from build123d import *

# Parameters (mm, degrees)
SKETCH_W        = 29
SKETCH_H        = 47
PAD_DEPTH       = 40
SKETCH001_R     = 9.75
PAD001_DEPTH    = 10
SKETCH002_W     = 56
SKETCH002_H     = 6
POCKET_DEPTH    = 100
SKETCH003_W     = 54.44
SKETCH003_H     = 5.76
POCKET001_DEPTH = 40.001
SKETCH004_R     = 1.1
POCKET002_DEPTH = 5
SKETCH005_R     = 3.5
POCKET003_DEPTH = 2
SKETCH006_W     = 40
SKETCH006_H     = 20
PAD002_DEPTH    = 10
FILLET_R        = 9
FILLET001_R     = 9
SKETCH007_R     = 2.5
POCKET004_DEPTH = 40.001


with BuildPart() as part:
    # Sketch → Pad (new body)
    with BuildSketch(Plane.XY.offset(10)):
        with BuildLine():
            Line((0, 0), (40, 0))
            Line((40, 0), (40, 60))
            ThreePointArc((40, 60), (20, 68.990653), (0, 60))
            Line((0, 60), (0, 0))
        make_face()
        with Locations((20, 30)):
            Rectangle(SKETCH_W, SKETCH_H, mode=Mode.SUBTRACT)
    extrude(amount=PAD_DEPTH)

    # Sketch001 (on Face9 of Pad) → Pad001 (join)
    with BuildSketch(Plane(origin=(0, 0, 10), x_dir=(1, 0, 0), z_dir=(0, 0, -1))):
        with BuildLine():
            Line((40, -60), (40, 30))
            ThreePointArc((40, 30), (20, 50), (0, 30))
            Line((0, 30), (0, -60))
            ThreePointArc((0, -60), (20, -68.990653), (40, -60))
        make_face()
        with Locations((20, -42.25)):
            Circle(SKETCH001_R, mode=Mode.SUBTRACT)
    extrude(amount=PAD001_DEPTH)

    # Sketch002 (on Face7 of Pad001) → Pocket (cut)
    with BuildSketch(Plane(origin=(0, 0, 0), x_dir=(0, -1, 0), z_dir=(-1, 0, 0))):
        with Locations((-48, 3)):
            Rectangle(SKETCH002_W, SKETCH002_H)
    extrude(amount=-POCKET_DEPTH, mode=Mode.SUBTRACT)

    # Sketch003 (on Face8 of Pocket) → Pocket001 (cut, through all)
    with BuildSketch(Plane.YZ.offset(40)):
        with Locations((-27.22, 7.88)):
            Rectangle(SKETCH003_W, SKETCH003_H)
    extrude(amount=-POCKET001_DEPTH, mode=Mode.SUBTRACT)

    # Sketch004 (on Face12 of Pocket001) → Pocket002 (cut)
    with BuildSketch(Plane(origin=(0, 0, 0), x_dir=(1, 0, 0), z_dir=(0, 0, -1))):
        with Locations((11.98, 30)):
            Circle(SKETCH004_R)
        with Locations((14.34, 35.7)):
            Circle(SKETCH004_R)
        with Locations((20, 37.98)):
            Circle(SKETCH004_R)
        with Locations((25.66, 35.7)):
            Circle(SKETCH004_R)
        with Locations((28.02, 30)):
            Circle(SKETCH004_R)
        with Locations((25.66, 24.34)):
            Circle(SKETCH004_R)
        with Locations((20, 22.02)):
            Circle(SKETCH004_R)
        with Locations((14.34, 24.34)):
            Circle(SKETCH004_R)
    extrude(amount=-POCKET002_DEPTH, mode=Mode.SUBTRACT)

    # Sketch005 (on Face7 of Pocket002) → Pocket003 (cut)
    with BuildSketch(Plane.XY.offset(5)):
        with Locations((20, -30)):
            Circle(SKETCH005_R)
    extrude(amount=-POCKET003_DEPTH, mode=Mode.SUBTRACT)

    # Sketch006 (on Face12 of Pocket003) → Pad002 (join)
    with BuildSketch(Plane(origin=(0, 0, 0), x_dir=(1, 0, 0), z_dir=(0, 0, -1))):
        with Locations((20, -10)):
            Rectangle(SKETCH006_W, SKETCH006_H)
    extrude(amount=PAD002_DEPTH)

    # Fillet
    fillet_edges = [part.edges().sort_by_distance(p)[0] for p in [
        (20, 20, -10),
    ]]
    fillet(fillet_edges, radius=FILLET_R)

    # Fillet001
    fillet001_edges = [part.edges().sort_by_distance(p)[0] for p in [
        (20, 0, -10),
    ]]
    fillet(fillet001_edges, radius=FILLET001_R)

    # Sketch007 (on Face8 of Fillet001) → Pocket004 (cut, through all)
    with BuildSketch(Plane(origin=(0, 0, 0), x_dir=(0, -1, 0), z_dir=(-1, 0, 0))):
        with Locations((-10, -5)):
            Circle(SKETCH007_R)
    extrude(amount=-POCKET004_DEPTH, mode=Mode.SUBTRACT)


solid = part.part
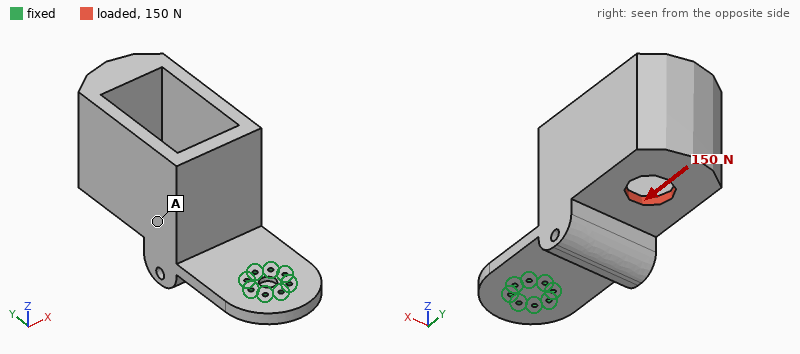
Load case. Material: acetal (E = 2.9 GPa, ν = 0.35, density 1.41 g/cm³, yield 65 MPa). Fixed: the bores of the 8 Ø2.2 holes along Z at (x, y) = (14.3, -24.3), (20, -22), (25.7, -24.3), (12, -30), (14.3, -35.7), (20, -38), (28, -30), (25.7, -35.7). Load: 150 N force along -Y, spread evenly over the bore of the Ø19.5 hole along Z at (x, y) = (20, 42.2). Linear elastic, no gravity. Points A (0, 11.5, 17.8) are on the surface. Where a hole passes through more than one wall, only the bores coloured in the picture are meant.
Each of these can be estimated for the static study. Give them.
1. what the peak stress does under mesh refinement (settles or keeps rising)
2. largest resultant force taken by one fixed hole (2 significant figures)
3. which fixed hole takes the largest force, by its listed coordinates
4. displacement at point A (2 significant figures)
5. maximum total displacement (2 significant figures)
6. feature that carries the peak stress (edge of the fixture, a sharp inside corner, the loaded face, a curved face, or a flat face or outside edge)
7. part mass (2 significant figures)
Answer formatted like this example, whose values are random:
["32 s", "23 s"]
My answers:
["keeps rising", "47 N", "(20, -22)", "0.46 mm", "1.5 mm", "edge of the fixture", "110 g"]
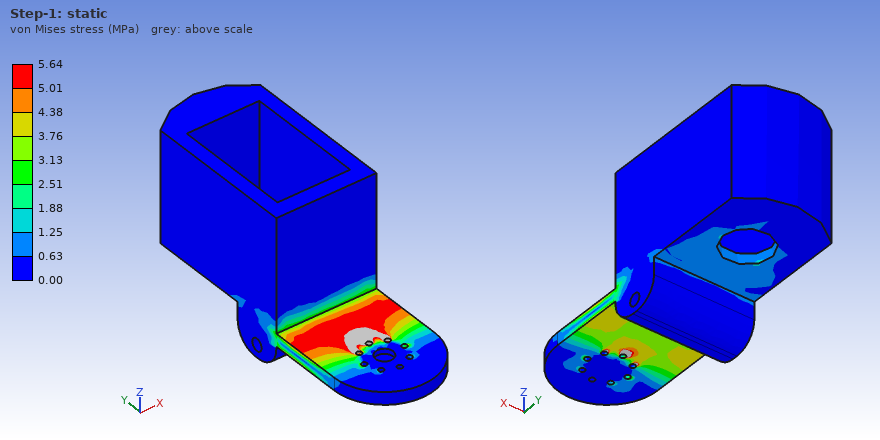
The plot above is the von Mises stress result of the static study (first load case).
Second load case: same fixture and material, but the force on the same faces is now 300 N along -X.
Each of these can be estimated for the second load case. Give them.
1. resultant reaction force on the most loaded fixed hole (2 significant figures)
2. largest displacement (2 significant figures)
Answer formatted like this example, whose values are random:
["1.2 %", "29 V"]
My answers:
["430 N", "1.6 mm"]
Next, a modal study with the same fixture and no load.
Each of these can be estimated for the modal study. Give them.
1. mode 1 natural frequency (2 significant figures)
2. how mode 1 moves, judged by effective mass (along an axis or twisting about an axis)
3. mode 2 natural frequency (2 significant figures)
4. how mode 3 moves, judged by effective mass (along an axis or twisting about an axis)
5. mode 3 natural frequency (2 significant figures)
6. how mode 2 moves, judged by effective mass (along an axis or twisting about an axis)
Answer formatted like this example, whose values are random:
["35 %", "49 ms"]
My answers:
["63 Hz", "along Z", "170 Hz", "along X", "500 Hz", "along X"]
